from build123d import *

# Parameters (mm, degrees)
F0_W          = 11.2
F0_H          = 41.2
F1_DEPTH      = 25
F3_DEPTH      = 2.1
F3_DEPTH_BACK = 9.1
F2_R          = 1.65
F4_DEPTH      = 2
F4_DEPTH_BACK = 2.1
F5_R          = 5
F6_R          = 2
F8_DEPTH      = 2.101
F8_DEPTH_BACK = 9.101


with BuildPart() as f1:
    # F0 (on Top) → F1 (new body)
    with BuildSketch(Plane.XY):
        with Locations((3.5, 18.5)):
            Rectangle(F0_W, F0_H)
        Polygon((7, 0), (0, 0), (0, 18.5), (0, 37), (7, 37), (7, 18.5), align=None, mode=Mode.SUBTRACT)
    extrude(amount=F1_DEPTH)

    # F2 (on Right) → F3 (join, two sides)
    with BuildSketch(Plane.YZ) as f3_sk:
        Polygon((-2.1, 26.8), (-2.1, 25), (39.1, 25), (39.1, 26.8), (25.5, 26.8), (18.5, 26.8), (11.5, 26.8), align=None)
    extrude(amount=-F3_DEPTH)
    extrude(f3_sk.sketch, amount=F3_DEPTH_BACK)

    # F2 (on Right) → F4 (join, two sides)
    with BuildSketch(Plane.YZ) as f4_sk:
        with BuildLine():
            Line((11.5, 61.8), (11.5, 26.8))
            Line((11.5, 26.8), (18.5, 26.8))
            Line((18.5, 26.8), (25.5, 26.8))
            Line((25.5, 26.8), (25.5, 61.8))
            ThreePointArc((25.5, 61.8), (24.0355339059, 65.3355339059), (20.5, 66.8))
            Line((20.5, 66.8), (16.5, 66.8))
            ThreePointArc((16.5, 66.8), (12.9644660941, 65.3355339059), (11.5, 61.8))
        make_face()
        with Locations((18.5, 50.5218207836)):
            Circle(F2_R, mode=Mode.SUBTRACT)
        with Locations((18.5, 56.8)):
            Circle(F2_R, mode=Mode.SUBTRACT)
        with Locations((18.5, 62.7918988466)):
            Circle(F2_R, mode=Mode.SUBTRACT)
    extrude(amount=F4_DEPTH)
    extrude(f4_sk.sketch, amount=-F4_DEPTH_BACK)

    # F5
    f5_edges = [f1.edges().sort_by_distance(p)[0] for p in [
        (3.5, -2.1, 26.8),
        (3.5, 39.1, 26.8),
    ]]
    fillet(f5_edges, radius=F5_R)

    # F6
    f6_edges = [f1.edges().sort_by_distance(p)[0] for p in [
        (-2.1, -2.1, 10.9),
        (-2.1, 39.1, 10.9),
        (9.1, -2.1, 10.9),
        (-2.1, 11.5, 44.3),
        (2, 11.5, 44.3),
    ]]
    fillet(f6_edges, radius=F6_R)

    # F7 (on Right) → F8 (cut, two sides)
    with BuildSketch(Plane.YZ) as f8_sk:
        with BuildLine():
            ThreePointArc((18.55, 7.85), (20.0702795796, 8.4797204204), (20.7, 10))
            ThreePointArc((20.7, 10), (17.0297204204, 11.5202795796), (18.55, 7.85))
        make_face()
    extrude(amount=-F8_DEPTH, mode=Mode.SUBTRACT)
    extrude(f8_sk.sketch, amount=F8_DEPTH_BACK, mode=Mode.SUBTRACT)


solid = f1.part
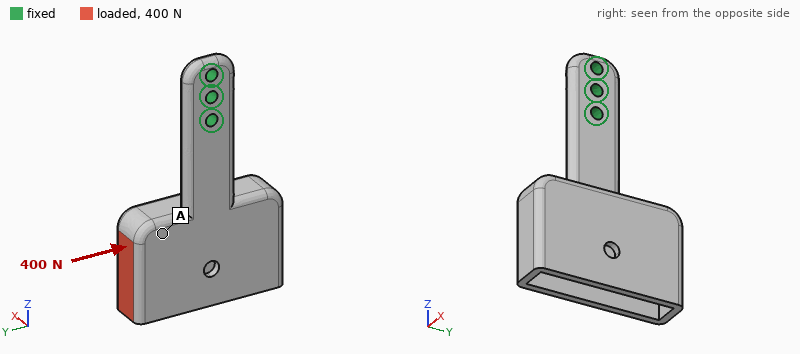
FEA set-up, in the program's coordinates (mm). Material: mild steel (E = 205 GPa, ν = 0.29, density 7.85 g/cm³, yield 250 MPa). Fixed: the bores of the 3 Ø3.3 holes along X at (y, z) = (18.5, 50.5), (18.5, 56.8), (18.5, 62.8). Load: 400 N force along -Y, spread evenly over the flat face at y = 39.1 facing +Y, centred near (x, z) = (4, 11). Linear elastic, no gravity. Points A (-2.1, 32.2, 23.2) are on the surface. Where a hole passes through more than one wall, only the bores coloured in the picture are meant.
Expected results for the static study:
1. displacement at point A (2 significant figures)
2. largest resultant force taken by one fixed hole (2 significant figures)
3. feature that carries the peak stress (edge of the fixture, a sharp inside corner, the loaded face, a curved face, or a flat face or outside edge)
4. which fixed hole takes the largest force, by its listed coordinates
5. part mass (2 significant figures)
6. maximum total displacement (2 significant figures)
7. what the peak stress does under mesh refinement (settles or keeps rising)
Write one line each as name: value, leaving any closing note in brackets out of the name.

displacement at point A: 0.056 mm
largest resultant force taken by one fixed hole: 1.4 kN
feature that carries the peak stress: edge of the fixture
which fixed hole takes the largest force, by its listed coordinates: (18.5, 50.5)
part mass: 59 g
maximum total displacement: 0.13 mm
what the peak stress does under mesh refinement: keeps rising
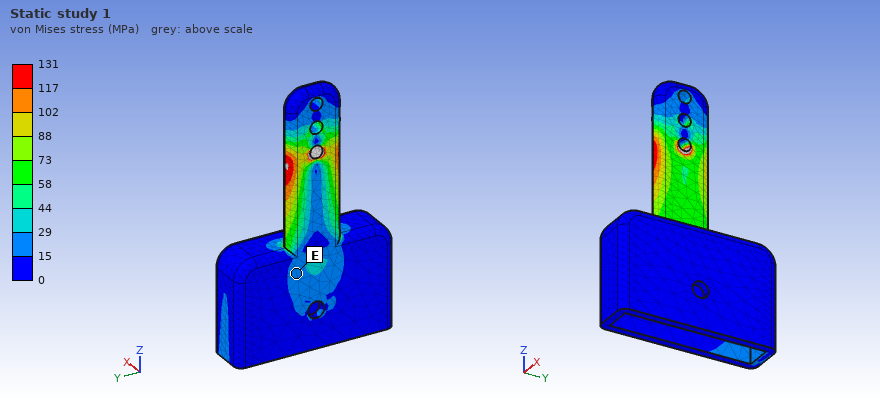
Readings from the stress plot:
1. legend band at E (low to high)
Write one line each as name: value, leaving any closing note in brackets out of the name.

legend band at E: 15 to 29 MPa
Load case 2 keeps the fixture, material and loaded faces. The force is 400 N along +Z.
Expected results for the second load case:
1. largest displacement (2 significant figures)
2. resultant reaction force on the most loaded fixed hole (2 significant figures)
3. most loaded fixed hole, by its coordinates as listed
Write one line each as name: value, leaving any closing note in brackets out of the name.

largest displacement: 0.15 mm
resultant reaction force on the most loaded fixed hole: 630 N
most loaded fixed hole, by its coordinates as listed: (18.5, 50.5)
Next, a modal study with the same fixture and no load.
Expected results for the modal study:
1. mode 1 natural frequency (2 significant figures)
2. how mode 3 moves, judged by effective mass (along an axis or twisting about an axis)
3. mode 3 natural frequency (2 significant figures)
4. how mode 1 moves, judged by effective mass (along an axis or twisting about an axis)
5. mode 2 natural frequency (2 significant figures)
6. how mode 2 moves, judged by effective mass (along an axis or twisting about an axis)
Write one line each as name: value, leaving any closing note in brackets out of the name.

mode 1 natural frequency: 670 Hz
how mode 3 moves, judged by effective mass: along Y
mode 3 natural frequency: 1800 Hz
how mode 1 moves, judged by effective mass: along X
mode 2 natural frequency: 1500 Hz
how mode 2 moves, judged by effective mass: along Y
